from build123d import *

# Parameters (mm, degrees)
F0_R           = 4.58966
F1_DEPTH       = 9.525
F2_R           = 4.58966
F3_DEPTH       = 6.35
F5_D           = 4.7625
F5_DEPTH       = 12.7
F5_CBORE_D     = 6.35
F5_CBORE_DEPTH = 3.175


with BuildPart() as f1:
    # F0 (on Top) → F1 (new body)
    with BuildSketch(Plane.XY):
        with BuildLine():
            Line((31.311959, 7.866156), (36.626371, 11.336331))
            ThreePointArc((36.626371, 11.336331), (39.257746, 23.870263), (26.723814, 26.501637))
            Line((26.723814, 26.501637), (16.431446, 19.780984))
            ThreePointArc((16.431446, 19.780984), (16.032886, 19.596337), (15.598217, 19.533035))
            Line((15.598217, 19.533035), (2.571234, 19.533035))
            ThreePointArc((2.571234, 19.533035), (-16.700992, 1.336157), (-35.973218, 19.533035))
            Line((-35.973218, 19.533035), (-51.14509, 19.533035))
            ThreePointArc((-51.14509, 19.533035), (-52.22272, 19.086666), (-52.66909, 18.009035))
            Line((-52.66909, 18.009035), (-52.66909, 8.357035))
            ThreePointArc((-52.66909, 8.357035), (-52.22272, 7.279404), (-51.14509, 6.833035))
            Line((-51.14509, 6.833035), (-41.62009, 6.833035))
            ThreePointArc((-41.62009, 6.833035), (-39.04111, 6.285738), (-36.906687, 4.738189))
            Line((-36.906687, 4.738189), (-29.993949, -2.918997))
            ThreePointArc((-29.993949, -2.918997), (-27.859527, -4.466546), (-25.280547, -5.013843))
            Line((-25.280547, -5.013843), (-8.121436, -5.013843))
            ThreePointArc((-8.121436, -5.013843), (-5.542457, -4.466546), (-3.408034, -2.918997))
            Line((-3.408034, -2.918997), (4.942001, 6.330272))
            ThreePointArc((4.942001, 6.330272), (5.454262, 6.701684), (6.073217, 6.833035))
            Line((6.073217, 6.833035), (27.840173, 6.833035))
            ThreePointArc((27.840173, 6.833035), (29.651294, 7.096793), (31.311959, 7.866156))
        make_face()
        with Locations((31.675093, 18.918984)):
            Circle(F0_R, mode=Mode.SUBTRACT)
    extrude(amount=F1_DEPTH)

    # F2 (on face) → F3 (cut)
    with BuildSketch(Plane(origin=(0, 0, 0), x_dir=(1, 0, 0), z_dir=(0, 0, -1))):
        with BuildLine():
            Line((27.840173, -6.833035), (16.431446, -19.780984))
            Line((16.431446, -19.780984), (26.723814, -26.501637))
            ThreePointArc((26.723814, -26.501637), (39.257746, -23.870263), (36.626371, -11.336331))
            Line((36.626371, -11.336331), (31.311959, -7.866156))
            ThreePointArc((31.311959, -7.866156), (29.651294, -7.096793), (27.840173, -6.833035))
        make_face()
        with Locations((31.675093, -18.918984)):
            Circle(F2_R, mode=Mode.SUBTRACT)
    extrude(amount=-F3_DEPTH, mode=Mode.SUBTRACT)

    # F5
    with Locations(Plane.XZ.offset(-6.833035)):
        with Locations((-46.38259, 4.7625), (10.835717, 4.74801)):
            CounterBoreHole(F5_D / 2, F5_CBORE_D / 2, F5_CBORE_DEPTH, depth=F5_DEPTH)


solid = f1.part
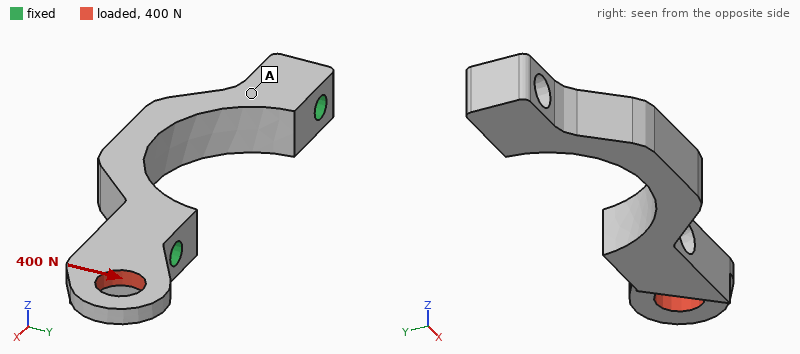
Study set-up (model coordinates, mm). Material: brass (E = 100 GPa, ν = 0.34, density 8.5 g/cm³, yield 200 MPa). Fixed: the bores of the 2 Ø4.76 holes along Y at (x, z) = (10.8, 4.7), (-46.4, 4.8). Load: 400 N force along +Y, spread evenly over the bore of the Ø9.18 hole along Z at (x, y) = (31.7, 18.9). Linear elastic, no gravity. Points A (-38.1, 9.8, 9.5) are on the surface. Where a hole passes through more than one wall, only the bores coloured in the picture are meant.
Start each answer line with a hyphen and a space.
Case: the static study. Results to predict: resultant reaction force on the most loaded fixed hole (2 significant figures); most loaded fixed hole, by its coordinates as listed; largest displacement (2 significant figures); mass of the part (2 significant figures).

- 400 N
- (10.8, 4.7)
- 31 µm
- 68 g
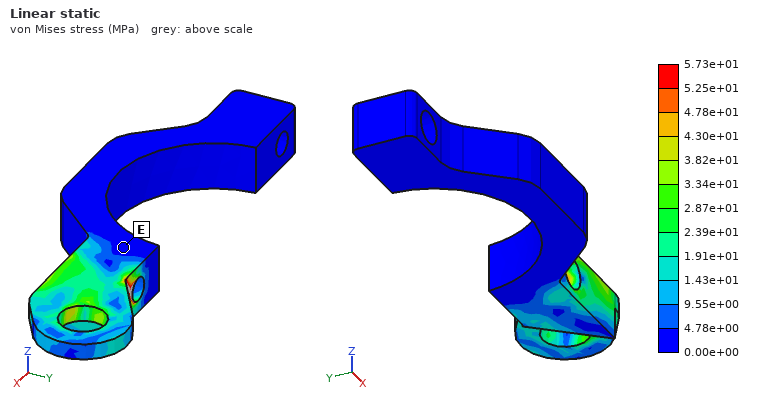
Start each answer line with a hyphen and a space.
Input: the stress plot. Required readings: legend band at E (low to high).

- 0.00e+00 to 4.78e+00 MPa
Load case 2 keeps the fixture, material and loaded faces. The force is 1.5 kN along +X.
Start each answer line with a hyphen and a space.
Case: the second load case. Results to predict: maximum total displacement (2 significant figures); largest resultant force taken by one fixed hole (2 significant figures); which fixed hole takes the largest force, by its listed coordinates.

- 43 µm
- 1.5 kN
- (10.8, 4.7)
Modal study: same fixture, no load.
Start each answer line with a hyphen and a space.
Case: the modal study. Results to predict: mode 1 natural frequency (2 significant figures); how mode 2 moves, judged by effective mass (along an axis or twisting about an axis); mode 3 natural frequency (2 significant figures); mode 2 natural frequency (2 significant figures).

- 4000 Hz
- along Z
- 8400 Hz
- 5800 Hz
